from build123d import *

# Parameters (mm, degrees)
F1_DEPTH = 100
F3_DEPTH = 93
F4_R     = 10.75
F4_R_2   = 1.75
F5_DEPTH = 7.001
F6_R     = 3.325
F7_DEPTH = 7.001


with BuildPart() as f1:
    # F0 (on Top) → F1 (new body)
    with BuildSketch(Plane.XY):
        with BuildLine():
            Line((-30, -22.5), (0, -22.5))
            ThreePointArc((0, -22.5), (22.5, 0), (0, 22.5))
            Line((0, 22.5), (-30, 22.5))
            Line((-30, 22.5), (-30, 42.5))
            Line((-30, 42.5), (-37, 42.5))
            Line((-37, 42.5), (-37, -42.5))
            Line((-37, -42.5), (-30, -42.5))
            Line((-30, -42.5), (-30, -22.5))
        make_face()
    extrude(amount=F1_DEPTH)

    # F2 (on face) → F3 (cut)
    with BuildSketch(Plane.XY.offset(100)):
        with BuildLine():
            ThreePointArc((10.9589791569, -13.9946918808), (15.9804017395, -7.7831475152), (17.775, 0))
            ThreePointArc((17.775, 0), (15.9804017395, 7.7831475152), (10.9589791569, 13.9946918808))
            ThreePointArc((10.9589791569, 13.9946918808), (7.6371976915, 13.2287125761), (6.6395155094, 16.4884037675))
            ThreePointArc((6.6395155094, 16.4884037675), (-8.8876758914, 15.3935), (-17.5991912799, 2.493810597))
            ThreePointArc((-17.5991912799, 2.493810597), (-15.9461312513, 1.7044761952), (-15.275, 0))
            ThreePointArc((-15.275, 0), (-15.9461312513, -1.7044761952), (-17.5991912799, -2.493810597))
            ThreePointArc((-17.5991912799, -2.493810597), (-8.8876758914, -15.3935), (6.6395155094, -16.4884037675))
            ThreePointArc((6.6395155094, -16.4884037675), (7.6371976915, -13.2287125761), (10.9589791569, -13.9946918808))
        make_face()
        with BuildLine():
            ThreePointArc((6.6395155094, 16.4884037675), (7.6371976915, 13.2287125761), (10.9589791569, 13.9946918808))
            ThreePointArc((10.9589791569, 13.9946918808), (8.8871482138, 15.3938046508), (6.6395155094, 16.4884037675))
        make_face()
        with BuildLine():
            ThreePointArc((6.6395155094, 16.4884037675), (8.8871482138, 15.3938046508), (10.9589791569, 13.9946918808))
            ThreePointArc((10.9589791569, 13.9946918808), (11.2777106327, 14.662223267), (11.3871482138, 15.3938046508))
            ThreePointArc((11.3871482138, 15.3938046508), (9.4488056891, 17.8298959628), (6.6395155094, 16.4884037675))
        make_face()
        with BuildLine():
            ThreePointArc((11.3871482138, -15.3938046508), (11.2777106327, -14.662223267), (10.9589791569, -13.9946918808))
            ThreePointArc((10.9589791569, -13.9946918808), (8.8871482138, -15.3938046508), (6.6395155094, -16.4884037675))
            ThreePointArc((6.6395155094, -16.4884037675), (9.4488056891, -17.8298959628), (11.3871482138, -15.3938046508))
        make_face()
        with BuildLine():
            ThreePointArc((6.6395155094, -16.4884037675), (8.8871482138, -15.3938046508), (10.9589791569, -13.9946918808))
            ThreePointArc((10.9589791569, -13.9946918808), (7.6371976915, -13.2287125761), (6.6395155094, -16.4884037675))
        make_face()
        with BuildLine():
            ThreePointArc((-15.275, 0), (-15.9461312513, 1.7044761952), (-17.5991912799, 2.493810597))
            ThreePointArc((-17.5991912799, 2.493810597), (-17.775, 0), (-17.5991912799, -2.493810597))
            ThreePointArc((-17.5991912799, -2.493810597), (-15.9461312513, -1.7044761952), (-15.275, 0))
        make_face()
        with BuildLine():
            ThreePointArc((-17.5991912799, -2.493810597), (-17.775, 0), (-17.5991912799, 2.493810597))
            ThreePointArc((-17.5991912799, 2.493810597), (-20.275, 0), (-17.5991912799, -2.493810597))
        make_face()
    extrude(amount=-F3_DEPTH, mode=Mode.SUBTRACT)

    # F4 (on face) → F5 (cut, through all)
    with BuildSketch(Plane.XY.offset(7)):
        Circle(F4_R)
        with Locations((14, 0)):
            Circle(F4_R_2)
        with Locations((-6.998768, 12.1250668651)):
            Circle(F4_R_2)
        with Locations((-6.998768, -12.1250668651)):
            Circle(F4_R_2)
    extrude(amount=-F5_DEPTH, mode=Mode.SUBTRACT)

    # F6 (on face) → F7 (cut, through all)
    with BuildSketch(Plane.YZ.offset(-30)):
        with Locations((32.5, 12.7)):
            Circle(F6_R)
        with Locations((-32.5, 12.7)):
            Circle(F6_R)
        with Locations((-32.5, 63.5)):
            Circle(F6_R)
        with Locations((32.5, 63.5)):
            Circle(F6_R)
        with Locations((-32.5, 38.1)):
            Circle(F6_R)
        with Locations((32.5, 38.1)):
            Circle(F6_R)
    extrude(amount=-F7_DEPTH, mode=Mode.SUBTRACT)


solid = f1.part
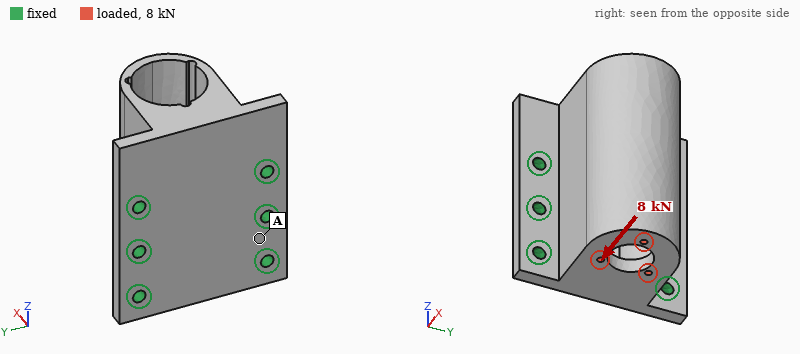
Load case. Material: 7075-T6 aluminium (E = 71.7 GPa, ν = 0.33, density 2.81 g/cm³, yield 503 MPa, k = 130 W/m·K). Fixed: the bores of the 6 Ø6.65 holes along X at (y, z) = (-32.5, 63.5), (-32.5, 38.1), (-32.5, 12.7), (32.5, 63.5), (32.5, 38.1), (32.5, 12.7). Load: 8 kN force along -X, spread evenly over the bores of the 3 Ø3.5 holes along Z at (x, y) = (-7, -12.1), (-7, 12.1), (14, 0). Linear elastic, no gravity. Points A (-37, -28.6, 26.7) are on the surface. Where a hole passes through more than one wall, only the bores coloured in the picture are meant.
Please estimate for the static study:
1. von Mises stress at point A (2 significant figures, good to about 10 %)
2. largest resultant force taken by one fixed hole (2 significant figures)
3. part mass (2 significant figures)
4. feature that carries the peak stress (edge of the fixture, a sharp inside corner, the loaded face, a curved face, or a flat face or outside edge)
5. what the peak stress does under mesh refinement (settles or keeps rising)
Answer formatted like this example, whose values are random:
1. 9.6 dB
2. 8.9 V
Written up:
1. 17 MPa
2. 4.2 kN
3. 490 g
4. edge of the fixture
5. keeps rising
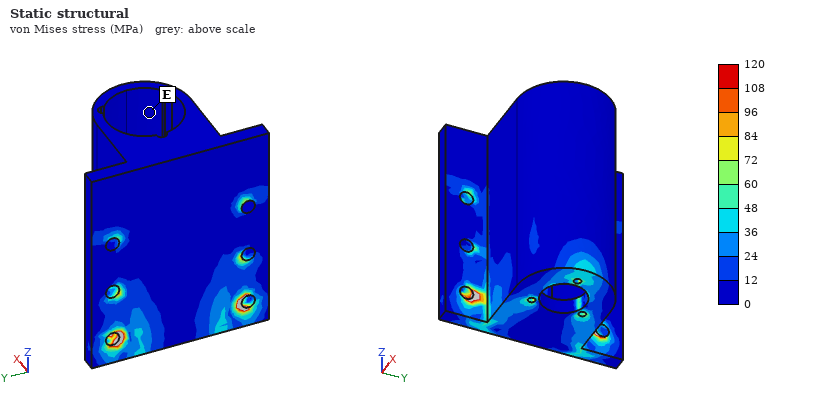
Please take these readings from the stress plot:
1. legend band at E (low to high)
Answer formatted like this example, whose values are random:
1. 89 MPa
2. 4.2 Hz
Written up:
1. 0 to 12 MPa
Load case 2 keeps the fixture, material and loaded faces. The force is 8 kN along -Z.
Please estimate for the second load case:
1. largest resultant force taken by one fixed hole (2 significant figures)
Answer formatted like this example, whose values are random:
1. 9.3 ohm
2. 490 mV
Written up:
1. 3.0 kN
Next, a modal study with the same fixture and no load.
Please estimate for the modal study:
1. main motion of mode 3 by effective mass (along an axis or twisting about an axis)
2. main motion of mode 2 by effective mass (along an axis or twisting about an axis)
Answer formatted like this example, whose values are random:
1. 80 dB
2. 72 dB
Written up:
1. along X
2. along Y
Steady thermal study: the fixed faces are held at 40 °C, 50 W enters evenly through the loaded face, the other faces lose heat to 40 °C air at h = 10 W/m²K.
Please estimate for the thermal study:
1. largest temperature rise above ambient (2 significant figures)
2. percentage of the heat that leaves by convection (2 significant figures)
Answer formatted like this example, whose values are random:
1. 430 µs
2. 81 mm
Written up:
1. 30 K
2. 5.7 %
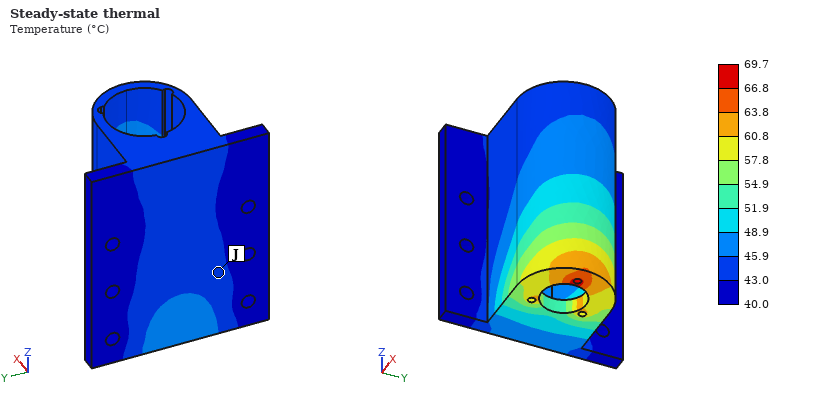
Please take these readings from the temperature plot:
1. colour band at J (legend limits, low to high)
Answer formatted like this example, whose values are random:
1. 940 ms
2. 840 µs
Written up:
1. 43.0 to 45.9 °C
